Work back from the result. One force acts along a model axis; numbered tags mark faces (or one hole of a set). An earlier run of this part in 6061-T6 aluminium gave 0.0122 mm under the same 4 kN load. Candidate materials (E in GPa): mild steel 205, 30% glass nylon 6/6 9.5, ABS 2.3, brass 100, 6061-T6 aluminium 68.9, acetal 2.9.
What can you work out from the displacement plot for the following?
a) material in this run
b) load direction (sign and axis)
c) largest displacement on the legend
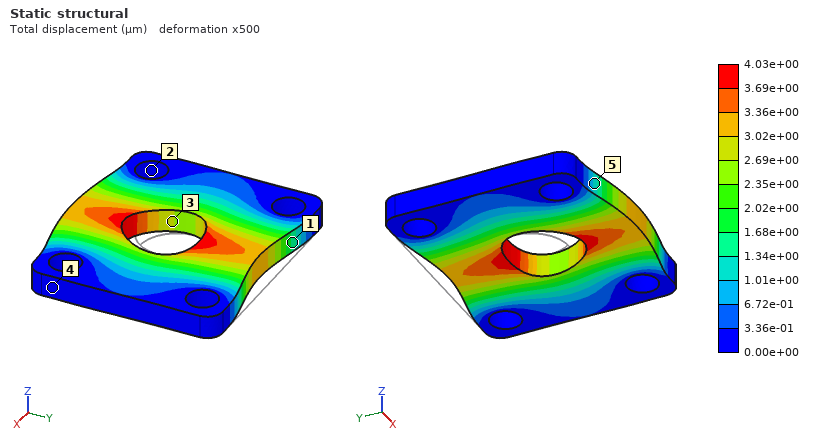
mild steel
-Y
4.03e+00 µm
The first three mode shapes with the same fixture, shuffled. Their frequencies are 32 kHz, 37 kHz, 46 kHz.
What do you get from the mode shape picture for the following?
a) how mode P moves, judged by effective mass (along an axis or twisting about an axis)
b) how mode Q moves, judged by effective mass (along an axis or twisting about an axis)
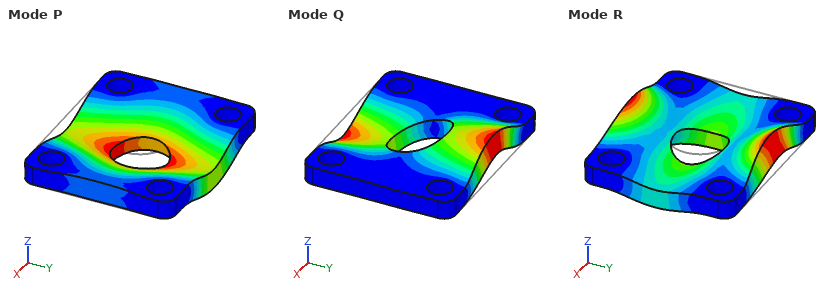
along Z
twisting about X
